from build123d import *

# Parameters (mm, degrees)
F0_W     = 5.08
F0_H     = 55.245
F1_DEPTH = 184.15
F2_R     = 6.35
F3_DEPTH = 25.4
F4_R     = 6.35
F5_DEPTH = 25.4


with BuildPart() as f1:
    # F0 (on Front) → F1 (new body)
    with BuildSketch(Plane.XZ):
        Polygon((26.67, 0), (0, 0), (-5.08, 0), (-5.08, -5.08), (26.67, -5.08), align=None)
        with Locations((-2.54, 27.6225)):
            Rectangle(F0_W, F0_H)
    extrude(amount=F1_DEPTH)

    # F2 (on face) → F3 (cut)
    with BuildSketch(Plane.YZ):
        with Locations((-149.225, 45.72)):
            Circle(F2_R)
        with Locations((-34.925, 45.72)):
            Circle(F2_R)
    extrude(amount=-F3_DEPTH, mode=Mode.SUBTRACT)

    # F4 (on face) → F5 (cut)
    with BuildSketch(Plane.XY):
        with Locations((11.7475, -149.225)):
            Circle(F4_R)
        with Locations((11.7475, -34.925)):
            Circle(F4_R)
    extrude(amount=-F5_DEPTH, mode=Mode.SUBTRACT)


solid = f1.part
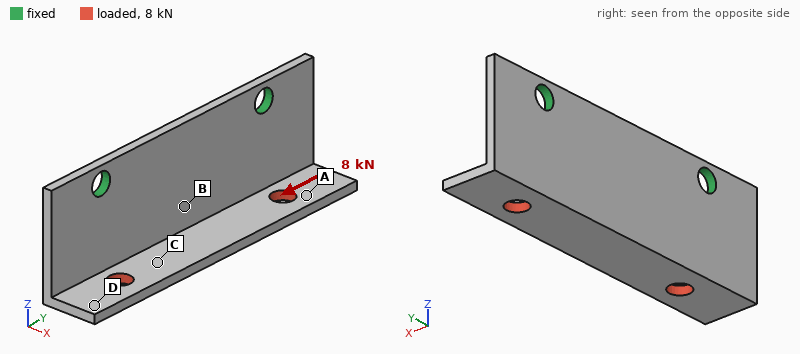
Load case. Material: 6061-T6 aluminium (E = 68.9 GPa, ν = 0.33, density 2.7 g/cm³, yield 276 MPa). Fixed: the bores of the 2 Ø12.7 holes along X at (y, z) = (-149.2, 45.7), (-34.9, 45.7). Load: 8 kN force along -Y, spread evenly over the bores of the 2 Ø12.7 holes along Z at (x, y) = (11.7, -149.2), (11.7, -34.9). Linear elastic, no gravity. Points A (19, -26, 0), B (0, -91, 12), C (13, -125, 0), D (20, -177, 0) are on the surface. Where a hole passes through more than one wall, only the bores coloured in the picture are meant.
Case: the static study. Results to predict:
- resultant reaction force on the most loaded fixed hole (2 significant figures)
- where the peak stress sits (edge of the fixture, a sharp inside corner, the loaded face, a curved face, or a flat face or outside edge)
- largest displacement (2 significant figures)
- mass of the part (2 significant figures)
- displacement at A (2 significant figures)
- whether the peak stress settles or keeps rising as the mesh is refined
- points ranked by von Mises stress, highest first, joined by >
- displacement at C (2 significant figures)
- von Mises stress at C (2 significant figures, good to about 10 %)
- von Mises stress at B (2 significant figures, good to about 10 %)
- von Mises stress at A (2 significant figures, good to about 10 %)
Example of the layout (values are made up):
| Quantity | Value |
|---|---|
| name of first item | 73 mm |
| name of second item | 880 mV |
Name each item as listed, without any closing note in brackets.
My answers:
| Quantity | Value |
|---|---|
| resultant reaction force on the most loaded fixed hole | 5.0 kN |
| where the peak stress sits | edge of the fixture |
| largest displacement | 0.72 mm |
| mass of the part | 210 g |
| displacement at A | 0.47 mm |
| whether the peak stress settles or keeps rising as the mesh is refined | keeps rising |
| points ranked by von Mises stress, highest first, joined by > | B > C > A > D |
| displacement at C | 0.25 mm |
| von Mises stress at C | 45 MPa |
| von Mises stress at B | 60 MPa |
| von Mises stress at A | 24 MPa |
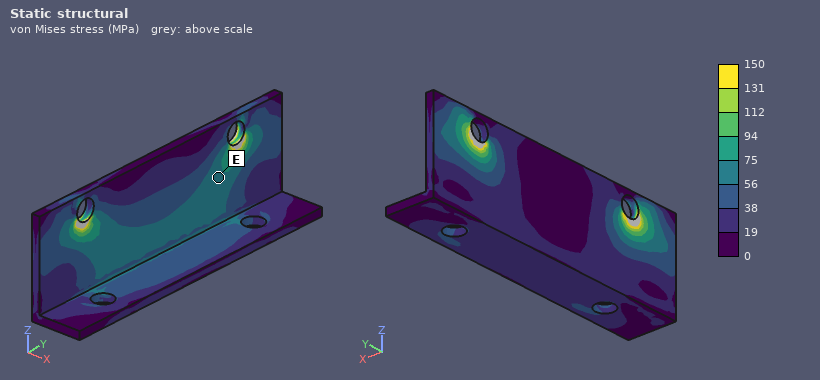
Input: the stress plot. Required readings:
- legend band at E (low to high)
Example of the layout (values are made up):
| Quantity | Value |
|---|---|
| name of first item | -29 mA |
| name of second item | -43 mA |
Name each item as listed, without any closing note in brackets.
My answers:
| Quantity | Value |
|---|---|
| legend band at E | 56 to 75 MPa |
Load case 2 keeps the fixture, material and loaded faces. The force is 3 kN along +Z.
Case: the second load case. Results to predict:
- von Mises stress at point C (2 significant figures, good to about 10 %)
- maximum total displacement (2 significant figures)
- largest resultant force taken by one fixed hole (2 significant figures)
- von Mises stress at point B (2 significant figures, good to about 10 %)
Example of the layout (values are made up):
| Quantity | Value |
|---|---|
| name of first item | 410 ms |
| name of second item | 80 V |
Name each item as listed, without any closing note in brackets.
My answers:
| Quantity | Value |
|---|---|
| von Mises stress at point C | 28 MPa |
| maximum total displacement | 0.72 mm |
| largest resultant force taken by one fixed hole | 1.5 kN |
| von Mises stress at point B | 30 MPa |
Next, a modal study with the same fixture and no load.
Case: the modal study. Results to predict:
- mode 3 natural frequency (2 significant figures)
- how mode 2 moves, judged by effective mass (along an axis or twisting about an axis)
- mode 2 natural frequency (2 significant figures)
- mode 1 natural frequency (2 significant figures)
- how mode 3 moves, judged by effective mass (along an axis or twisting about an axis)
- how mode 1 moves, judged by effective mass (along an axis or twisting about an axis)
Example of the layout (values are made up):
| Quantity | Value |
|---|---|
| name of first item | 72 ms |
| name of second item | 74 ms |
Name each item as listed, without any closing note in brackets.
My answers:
| Quantity | Value |
|---|---|
| mode 3 natural frequency | 2500 Hz |
| how mode 2 moves, judged by effective mass | twisting about Z |
| mode 2 natural frequency | 1200 Hz |
| mode 1 natural frequency | 810 Hz |
| how mode 3 moves, judged by effective mass | along X |
| how mode 1 moves, judged by effective mass | along X |
